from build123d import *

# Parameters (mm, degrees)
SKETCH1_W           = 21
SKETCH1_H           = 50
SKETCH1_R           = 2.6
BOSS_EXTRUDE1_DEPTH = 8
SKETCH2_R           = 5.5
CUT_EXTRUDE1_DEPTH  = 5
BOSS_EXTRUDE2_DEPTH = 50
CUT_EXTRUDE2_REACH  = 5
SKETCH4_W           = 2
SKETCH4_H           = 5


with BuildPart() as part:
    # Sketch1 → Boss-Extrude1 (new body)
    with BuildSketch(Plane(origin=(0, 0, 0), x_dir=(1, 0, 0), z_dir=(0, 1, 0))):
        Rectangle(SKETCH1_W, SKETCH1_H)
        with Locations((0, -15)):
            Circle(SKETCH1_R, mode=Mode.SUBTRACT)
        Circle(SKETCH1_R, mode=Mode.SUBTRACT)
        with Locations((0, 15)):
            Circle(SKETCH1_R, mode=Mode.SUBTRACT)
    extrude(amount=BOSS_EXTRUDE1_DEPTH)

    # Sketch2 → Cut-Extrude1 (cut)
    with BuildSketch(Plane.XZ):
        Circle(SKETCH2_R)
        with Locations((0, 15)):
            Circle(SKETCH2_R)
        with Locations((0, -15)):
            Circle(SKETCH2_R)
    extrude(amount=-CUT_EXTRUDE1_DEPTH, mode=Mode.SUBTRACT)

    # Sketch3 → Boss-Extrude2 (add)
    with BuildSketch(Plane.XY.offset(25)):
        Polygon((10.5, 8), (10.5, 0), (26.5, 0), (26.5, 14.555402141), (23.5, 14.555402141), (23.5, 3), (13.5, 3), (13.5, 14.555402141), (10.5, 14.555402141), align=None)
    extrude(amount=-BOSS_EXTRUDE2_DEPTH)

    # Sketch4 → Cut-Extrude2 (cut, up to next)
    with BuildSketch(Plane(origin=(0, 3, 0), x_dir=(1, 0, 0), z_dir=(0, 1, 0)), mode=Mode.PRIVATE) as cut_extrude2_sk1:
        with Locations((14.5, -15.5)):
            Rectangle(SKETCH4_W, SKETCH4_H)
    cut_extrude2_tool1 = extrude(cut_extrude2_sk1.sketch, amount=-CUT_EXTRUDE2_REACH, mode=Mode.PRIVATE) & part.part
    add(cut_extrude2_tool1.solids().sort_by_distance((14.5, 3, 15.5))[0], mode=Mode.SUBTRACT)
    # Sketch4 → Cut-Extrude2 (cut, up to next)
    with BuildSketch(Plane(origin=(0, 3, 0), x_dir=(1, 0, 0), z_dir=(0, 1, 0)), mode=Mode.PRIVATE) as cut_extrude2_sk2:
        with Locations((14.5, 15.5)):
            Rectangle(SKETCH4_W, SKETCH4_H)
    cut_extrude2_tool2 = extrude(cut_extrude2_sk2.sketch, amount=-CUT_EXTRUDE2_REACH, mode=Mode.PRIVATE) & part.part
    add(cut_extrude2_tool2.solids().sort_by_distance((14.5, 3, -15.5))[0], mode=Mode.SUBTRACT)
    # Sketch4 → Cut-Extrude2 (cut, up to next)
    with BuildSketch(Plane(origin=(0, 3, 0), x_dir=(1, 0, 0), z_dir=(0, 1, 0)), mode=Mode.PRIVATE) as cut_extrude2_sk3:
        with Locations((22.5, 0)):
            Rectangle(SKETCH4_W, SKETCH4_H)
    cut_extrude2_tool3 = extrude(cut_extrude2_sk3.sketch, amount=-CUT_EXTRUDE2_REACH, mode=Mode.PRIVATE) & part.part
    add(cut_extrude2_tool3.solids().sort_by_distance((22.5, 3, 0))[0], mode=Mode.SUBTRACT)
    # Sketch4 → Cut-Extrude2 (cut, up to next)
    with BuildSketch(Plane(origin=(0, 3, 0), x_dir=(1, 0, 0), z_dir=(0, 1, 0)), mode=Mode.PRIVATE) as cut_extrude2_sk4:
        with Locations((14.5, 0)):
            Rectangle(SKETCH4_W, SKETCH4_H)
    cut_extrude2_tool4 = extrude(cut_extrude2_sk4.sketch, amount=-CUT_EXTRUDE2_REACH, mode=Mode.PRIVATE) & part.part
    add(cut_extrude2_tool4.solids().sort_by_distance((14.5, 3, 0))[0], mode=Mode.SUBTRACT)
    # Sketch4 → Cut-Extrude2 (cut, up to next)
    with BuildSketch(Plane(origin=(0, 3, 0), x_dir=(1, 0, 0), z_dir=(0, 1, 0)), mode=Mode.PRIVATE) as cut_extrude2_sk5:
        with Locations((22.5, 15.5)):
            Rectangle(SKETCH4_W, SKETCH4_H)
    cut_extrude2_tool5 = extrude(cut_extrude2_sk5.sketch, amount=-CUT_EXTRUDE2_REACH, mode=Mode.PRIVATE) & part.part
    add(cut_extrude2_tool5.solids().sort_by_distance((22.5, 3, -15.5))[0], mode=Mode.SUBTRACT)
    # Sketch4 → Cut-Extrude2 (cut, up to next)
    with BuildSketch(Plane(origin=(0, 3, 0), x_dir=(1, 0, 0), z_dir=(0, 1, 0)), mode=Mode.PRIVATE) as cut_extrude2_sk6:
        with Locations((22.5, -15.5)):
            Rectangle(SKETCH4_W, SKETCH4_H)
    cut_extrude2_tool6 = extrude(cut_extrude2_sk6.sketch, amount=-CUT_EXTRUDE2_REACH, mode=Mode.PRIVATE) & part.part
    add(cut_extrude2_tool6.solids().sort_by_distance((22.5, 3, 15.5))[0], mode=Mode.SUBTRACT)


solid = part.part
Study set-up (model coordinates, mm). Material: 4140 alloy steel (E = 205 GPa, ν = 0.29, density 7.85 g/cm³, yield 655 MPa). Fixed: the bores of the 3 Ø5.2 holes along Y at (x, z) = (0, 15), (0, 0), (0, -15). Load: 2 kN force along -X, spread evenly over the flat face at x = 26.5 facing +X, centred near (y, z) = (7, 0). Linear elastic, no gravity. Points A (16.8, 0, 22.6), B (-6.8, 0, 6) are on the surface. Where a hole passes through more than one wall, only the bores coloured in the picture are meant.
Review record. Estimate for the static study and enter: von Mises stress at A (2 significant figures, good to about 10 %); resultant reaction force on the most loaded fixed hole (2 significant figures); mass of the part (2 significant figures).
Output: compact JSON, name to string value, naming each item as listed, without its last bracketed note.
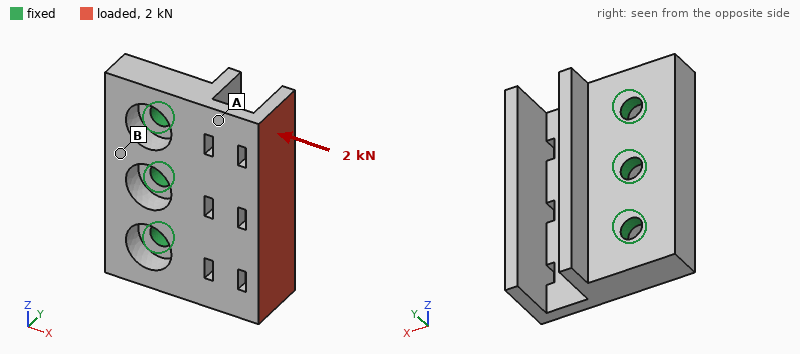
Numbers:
{"von Mises stress at A": "180 MPa", "resultant reaction force on the most loaded fixed hole": "720 N", "mass of the part": "98 g"}
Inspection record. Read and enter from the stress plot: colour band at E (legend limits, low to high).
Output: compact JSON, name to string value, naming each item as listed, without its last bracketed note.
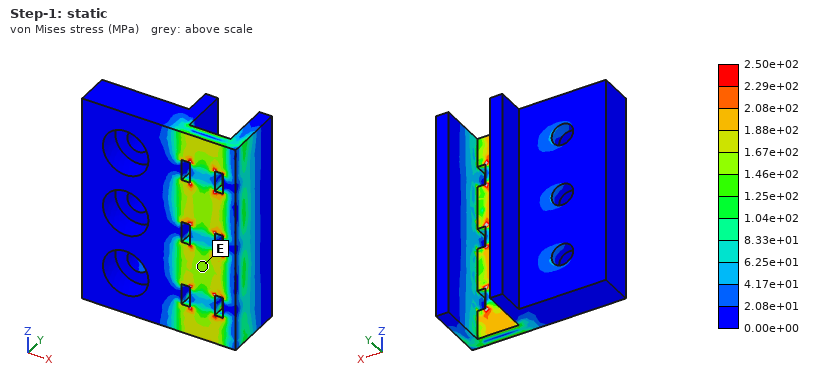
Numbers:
{"colour band at E": "1.46e+02 to 1.67e+02 MPa"}
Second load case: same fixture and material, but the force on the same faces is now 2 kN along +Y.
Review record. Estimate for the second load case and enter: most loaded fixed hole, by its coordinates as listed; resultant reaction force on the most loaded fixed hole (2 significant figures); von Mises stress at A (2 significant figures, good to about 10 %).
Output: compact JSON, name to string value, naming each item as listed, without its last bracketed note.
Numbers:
{"most loaded fixed hole, by its coordinates as listed": "(0, 0)", "resultant reaction force on the most loaded fixed hole": "800 N", "von Mises stress at A": "320 MPa"}
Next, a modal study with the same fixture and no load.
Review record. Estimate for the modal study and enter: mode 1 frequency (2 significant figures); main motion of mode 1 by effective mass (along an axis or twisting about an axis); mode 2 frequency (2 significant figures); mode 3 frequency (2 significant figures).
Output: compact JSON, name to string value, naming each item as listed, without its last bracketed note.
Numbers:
{"mode 1 frequency": "3500 Hz", "main motion of mode 1 by effective mass": "along Y", "mode 2 frequency": "5600 Hz", "mode 3 frequency": "7400 Hz"}
